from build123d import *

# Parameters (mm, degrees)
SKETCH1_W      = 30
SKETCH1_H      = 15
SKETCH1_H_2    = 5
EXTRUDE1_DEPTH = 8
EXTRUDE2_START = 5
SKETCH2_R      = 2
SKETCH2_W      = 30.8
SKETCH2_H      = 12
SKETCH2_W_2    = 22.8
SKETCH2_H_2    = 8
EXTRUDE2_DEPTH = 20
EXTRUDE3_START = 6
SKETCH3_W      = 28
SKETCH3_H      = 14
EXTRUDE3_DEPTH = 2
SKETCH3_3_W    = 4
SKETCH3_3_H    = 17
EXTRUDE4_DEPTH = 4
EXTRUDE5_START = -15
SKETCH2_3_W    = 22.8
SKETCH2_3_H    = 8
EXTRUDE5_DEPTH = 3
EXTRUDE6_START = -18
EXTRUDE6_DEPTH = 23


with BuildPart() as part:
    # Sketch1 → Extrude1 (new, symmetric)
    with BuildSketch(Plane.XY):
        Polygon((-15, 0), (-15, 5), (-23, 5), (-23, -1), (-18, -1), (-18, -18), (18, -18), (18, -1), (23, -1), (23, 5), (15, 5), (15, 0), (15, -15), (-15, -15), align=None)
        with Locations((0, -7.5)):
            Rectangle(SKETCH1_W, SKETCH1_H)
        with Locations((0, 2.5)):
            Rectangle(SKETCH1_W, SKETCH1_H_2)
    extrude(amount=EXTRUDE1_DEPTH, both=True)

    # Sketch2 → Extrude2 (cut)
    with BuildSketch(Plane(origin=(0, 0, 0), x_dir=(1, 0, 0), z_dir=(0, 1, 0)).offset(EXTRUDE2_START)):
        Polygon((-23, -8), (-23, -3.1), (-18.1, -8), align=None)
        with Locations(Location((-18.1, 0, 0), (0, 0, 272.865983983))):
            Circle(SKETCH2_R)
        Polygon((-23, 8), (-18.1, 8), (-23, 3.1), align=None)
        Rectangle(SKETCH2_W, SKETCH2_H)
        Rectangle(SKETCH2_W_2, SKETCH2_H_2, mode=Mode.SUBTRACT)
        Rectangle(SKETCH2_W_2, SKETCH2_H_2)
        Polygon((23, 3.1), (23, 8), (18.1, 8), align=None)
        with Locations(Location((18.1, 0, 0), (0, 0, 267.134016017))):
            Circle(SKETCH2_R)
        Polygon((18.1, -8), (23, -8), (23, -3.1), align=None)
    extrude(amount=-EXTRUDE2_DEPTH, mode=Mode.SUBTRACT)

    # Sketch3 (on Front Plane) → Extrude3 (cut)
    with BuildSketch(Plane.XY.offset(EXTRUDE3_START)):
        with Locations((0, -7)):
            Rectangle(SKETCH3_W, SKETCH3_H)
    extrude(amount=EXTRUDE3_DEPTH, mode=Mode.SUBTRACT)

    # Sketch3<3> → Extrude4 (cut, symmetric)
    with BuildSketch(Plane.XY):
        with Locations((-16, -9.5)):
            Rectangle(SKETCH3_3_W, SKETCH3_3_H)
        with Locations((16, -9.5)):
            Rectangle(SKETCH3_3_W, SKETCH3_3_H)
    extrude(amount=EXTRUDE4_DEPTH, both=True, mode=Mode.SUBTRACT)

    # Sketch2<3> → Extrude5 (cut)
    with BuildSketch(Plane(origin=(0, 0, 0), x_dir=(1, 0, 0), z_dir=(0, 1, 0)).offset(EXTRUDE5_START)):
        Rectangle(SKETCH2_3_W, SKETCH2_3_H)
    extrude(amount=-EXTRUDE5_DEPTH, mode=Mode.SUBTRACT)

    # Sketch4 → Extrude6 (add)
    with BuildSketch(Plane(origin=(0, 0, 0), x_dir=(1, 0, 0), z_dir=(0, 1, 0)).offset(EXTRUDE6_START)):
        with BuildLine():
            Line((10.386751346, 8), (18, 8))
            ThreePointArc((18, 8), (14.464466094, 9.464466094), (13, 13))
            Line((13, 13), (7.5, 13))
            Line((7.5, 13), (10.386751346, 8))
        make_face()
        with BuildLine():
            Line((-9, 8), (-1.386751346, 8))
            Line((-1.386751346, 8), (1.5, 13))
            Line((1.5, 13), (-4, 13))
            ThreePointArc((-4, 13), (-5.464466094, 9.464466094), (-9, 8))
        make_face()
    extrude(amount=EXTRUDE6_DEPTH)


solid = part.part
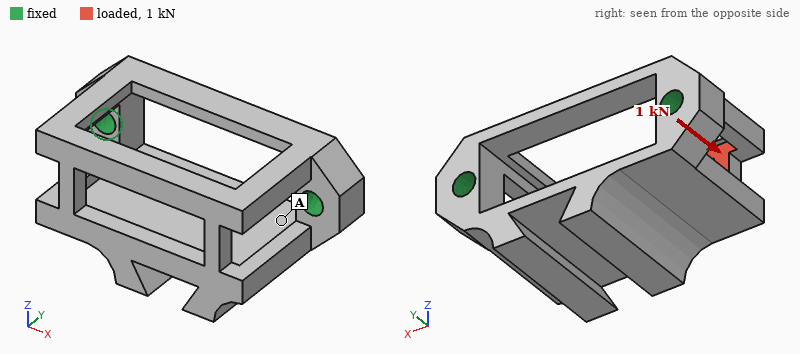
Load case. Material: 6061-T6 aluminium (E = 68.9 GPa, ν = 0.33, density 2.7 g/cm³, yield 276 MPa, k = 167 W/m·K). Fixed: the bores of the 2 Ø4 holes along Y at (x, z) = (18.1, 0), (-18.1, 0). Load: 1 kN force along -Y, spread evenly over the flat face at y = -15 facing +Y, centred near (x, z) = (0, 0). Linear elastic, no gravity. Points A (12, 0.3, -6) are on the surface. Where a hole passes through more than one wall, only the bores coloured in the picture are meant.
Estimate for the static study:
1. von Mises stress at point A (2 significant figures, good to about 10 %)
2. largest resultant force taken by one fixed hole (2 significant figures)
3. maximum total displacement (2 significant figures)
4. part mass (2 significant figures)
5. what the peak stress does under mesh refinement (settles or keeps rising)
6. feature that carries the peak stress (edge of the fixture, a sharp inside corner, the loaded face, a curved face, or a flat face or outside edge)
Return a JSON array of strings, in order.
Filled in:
["16 MPa", "510 N", "72 µm", "15 g", "keeps rising", "a sharp inside corner"]
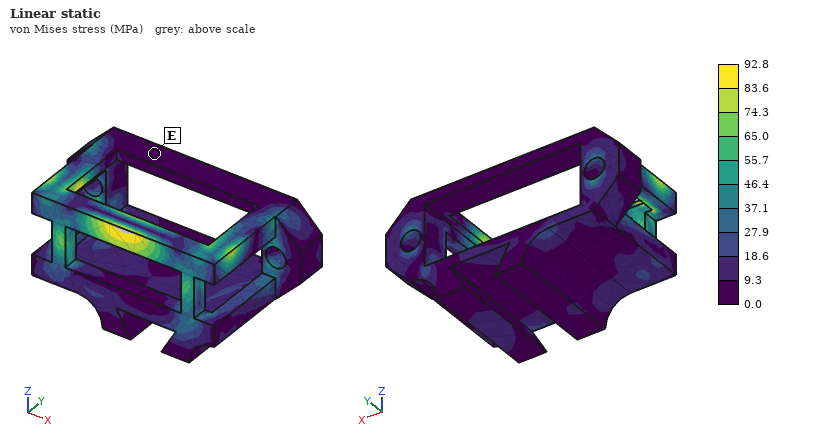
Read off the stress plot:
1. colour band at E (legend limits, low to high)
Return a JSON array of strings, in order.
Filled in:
["0.0 to 9.3 MPa"]
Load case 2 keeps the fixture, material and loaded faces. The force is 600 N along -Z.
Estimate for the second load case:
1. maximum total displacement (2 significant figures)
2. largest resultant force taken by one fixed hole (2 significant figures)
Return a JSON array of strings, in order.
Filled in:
["0.14 mm", "310 N"]
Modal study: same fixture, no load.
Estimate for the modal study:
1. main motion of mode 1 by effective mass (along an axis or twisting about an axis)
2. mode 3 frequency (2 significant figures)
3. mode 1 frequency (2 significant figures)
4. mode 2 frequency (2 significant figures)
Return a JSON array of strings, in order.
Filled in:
["along Z", "8500 Hz", "4700 Hz", "7900 Hz"]
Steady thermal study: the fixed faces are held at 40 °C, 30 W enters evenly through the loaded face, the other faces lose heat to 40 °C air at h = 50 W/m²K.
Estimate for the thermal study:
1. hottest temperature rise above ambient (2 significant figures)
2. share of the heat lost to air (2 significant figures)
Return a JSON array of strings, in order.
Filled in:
["56 K", "16 %"]
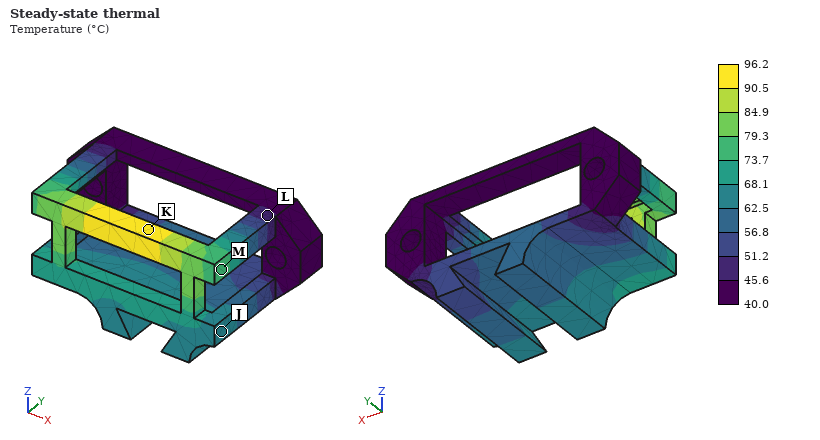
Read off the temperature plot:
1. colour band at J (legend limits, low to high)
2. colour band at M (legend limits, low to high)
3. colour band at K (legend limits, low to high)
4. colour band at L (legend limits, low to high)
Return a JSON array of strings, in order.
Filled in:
["62.5 to 68.1 °C", "73.7 to 79.3 °C", "90.5 to 96.2 °C", "45.6 to 51.2 °C"]
